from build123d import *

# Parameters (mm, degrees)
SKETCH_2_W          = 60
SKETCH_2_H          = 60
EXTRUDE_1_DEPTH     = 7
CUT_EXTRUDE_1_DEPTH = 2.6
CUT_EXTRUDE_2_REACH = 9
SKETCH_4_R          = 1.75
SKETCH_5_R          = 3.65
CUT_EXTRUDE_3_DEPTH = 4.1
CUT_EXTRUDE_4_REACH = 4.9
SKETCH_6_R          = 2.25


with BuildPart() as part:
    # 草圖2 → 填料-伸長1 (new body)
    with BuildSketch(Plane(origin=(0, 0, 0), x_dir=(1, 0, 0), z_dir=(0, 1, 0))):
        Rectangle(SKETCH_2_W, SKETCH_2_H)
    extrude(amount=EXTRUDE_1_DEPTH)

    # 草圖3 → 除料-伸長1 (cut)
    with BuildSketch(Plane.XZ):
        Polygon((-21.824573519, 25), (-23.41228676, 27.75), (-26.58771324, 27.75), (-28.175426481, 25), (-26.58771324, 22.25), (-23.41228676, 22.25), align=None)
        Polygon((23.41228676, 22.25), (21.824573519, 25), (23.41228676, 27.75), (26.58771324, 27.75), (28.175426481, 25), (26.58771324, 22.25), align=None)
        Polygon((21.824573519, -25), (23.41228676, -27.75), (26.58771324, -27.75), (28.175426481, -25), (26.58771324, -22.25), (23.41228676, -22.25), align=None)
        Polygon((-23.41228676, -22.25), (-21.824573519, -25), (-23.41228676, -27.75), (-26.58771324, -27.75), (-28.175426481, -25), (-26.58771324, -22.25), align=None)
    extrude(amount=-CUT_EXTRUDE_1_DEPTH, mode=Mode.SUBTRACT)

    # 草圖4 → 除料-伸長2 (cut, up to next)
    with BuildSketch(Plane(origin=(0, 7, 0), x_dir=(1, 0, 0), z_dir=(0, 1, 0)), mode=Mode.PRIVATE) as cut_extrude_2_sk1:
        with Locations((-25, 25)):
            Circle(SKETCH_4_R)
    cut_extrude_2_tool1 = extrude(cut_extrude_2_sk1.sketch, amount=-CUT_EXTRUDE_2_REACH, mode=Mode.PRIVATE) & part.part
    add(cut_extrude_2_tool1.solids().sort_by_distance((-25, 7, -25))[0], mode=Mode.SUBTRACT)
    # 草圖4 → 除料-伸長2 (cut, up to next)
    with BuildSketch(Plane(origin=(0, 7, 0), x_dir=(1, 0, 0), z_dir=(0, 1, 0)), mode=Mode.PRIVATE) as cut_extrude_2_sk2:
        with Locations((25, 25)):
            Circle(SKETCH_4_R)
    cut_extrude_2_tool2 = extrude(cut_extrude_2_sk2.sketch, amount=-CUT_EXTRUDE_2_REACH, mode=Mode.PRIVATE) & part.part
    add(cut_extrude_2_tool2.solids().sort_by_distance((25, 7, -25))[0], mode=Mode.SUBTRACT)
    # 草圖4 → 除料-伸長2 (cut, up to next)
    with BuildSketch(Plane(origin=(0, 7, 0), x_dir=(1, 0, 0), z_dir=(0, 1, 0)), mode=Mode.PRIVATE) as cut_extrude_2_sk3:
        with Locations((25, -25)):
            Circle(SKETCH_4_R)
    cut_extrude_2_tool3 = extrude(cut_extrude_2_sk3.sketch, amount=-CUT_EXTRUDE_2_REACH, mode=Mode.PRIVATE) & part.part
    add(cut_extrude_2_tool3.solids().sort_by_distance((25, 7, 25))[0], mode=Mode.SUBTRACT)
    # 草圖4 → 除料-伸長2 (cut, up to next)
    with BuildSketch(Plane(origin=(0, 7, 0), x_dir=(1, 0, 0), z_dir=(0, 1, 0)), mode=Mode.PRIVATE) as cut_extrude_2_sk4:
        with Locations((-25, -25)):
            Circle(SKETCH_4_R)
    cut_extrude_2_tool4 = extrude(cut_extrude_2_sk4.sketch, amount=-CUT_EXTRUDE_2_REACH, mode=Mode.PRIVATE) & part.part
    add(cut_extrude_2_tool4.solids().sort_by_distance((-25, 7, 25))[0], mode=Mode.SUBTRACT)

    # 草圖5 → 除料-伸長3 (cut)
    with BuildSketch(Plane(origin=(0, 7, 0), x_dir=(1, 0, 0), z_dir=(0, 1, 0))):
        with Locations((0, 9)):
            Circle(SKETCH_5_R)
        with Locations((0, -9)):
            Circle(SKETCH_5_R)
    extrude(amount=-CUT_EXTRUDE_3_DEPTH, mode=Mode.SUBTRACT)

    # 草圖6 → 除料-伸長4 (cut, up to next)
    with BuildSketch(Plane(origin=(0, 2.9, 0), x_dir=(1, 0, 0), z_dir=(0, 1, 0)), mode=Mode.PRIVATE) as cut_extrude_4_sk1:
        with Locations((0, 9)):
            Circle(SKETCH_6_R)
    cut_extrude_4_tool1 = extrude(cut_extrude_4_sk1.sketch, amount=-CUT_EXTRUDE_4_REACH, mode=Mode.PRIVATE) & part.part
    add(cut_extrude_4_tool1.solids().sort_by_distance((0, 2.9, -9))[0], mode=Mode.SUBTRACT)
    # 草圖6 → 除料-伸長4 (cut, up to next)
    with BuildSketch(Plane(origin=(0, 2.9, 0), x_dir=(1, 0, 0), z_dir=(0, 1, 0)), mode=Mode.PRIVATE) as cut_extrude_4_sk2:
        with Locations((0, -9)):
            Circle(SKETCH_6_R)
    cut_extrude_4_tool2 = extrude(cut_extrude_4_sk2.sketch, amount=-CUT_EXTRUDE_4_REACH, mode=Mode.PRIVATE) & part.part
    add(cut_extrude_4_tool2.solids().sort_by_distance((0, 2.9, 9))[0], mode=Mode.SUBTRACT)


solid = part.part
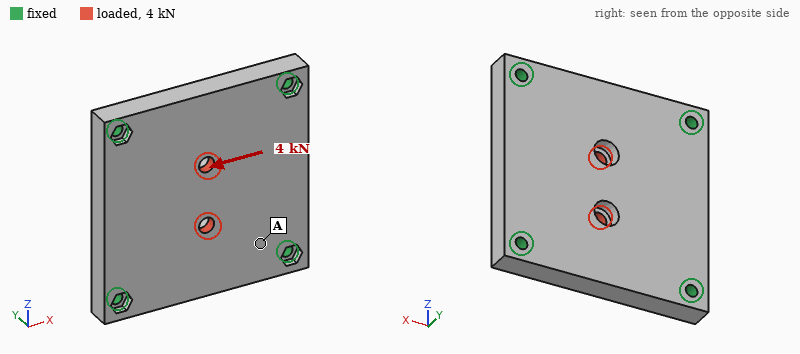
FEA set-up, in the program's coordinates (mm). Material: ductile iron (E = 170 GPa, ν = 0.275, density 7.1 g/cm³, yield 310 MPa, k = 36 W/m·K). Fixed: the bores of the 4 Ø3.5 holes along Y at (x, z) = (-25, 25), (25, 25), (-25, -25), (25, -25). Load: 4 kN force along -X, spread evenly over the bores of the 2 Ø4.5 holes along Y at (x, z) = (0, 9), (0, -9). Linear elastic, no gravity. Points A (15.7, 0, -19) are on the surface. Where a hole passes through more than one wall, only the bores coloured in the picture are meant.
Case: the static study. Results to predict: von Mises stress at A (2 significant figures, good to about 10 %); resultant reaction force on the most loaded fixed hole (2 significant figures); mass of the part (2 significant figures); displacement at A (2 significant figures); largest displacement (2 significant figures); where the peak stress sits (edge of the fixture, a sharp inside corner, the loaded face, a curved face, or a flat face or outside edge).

11 MPa
1.1 kN
170 g
1.1 µm
3.6 µm
a sharp inside corner
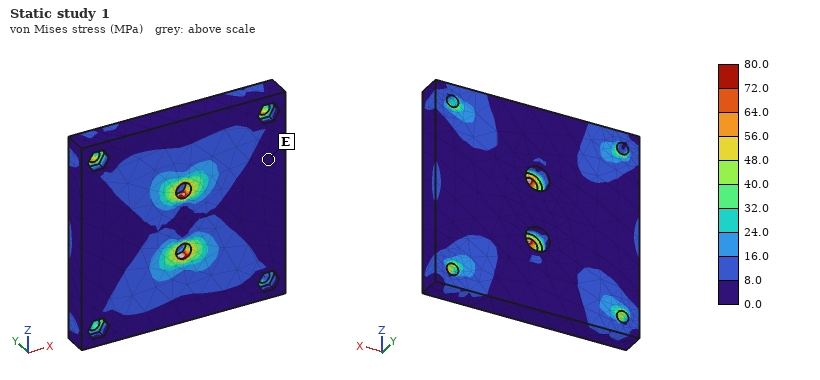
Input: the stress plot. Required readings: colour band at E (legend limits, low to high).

0.0 to 8.0 MPa
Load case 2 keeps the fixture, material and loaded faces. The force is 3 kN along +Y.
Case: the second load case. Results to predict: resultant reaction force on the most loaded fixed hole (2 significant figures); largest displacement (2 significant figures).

1.1 kN
30 µm
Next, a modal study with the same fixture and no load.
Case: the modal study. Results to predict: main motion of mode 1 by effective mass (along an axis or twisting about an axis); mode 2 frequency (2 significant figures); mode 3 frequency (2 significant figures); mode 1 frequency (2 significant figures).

along Y
12 kHz
12 kHz
7100 Hz
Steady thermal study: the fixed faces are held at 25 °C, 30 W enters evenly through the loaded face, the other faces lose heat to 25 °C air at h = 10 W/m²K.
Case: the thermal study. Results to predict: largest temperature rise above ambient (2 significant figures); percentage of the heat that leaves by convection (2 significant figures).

62 K
6.6 %
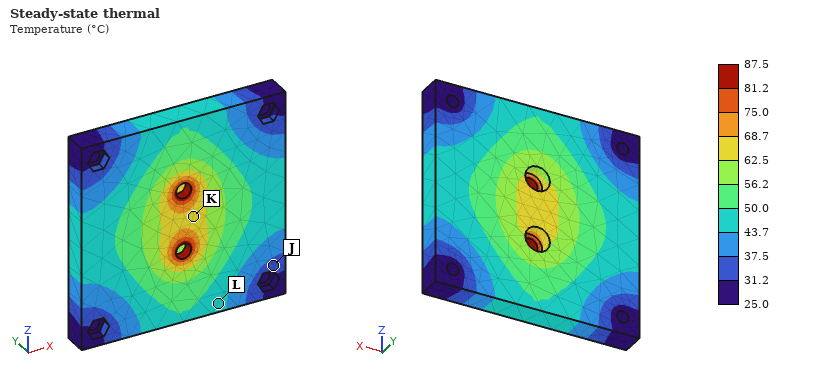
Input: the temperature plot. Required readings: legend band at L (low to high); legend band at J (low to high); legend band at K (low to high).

43.7 to 50.0 °C
31.2 to 37.5 °C
62.5 to 68.7 °C
